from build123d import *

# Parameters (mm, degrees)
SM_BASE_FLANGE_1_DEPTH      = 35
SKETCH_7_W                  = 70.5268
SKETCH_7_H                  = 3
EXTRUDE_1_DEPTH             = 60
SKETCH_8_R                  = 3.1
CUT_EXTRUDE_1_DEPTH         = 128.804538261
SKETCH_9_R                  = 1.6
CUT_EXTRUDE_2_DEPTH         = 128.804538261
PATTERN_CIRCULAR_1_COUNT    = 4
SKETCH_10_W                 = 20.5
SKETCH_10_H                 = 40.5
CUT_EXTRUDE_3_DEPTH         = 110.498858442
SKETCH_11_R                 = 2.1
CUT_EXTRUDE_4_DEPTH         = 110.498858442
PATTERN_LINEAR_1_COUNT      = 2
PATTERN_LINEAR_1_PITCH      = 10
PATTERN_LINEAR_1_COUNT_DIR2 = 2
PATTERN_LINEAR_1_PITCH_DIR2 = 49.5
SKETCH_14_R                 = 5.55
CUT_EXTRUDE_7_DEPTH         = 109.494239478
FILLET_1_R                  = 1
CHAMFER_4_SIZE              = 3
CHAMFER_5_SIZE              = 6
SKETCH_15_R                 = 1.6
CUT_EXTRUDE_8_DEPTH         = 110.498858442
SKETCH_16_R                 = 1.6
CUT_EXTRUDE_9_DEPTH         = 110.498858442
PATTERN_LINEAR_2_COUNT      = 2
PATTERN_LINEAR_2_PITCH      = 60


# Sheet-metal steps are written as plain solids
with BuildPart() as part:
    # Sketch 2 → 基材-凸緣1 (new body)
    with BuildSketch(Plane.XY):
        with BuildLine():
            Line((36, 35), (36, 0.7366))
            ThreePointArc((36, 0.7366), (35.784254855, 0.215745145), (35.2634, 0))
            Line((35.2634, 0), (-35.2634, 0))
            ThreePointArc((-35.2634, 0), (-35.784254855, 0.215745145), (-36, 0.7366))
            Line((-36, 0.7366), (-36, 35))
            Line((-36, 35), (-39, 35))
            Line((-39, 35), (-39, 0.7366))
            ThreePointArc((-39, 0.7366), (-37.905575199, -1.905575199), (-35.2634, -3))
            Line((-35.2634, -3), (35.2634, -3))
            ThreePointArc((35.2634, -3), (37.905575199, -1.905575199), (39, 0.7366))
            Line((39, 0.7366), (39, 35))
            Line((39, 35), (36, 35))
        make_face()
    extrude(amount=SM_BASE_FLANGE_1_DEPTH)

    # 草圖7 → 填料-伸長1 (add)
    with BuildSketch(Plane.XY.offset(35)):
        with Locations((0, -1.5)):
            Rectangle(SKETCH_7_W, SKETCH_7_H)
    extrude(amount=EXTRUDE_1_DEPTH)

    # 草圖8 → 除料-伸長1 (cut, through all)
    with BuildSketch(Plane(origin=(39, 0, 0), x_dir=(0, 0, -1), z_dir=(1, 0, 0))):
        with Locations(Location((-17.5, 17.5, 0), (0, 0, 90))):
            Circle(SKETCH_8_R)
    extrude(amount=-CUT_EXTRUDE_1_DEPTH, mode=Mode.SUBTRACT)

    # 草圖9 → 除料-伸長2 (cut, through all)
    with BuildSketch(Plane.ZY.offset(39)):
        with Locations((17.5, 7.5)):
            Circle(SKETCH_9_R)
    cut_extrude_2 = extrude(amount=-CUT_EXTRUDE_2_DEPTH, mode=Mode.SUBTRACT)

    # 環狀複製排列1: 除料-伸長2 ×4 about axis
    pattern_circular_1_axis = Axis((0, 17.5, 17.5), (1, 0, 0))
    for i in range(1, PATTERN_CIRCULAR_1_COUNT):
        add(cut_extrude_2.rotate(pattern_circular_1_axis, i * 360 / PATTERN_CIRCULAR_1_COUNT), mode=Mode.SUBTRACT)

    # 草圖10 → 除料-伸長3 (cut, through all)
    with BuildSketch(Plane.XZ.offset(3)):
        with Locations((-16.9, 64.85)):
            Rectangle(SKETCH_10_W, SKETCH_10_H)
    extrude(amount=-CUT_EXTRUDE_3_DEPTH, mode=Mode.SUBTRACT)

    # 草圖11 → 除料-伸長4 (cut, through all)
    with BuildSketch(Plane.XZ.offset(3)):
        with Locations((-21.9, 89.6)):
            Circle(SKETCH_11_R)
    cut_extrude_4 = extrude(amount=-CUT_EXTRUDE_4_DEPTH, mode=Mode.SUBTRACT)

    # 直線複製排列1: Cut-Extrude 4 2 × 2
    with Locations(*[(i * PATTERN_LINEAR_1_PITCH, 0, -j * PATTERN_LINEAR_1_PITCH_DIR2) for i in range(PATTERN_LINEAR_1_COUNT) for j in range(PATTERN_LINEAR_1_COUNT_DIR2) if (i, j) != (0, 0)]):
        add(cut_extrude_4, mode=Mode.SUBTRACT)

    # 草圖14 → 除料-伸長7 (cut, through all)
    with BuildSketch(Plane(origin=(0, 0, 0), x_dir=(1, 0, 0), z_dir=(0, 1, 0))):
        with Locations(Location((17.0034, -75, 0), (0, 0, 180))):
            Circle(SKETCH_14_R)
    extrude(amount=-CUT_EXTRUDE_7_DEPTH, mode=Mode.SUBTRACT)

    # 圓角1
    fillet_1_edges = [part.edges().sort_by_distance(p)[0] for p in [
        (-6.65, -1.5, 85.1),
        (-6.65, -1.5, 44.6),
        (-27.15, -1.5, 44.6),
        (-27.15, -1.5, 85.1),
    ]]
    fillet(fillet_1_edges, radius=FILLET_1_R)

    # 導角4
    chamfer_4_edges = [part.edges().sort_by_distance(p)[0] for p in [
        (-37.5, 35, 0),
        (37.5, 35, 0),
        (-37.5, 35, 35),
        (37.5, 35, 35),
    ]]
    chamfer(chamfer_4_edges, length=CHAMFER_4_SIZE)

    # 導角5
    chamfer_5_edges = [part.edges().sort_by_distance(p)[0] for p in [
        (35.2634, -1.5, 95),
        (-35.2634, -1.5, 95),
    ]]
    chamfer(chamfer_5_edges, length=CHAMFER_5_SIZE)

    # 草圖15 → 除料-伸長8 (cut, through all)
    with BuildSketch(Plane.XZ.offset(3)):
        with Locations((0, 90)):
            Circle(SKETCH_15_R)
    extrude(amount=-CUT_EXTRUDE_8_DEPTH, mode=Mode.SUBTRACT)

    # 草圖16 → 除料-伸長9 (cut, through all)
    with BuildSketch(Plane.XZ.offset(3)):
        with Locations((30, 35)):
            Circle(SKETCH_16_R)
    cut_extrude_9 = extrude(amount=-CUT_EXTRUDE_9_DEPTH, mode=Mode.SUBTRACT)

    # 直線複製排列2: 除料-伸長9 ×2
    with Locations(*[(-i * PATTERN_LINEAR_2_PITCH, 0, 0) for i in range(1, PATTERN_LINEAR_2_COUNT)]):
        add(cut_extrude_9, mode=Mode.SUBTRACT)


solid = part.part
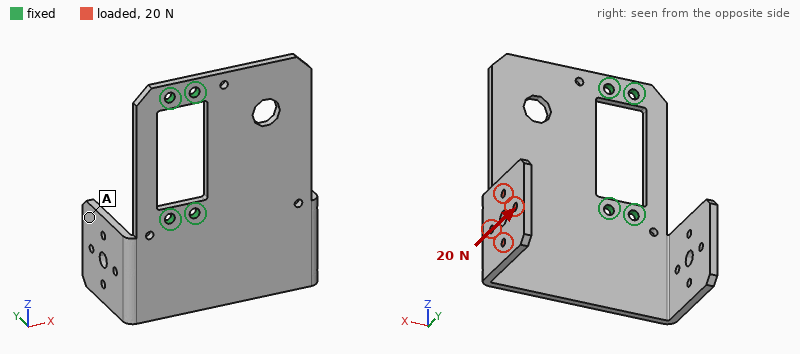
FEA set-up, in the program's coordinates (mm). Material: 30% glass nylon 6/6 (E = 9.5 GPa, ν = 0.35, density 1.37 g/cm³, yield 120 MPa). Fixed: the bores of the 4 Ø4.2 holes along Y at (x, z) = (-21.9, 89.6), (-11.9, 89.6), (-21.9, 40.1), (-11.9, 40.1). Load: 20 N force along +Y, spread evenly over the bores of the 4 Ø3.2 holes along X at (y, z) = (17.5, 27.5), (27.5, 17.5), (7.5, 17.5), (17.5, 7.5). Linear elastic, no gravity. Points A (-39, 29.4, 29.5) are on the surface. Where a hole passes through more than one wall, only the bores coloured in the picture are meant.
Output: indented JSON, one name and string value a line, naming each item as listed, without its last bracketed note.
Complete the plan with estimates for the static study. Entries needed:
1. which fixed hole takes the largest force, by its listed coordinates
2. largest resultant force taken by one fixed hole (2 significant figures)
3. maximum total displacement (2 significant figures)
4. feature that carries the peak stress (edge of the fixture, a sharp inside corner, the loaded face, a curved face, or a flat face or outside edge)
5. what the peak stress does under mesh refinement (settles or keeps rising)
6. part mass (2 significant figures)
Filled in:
{
  "which fixed hole takes the largest force, by its listed coordinates": "(-11.9, 40.1)",
  "largest resultant force taken by one fixed hole": "55 N",
  "maximum total displacement": "1.4 mm",
  "feature that carries the peak stress": "edge of the fixture",
  "what the peak stress does under mesh refinement": "keeps rising",
  "part mass": "34 g"
}
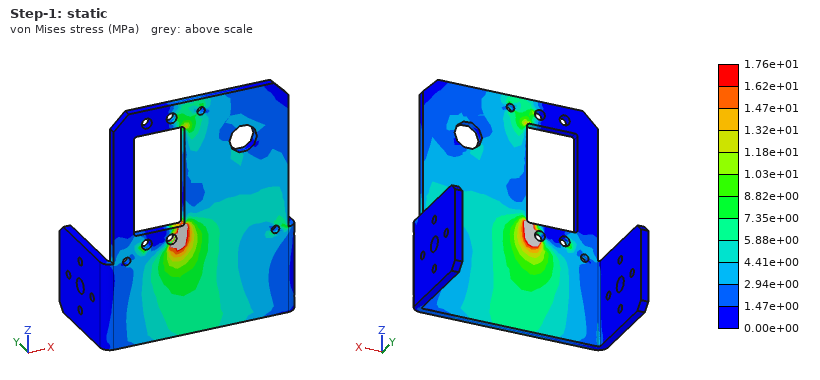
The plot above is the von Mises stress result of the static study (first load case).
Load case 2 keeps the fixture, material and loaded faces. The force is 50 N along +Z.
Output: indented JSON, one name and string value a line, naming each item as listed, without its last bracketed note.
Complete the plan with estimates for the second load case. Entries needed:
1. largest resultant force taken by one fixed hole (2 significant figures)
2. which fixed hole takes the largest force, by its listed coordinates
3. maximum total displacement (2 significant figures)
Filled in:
{
  "largest resultant force taken by one fixed hole": "60 N",
  "which fixed hole takes the largest force, by its listed coordinates": "(-11.9, 40.1)",
  "maximum total displacement": "1.4 mm"
}
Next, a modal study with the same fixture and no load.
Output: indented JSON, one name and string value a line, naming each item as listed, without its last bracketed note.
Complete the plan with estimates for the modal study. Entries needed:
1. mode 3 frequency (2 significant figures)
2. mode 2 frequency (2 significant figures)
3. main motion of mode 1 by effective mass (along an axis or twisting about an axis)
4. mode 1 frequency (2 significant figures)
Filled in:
{
  "mode 3 frequency": "470 Hz",
  "mode 2 frequency": "400 Hz",
  "main motion of mode 1 by effective mass": "along Y",
  "mode 1 frequency": "240 Hz"
}
